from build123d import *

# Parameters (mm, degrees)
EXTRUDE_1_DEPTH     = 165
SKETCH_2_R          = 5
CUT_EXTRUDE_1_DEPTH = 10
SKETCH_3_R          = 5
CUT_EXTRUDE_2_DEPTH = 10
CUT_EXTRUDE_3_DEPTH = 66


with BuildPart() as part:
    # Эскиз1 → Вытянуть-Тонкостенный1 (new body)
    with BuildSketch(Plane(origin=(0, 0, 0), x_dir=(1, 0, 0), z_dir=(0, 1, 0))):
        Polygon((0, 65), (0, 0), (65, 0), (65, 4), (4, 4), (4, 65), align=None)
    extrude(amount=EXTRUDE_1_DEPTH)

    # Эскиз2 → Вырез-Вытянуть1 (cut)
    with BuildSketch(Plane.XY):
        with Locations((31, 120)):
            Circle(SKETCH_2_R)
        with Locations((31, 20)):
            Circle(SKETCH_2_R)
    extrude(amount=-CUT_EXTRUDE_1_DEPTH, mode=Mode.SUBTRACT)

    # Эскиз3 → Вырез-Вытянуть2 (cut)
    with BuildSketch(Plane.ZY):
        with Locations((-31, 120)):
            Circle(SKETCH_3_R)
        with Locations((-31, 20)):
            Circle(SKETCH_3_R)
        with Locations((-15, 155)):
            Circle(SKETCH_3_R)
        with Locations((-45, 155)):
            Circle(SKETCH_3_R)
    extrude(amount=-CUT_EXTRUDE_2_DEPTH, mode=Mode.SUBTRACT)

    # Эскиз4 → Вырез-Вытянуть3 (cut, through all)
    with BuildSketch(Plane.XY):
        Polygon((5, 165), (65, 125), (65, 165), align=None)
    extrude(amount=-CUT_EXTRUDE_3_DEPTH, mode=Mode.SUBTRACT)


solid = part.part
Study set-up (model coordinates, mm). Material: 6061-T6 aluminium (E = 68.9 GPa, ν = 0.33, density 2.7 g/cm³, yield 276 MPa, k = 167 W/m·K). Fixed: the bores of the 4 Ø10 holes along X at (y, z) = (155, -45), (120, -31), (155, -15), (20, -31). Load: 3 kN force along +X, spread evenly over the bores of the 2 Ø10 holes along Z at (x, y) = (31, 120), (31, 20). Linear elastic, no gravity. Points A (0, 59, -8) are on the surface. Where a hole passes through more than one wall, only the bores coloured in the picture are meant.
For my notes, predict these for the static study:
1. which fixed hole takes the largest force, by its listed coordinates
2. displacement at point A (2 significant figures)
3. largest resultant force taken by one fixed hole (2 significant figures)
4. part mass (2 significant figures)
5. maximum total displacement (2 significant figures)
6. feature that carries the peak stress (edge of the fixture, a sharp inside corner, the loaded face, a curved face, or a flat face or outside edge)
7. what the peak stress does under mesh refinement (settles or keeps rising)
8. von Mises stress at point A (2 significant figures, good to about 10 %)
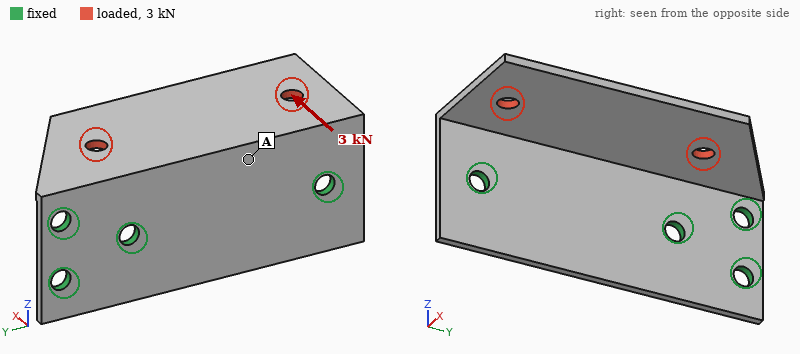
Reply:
(20, -31)
0.30 mm
1.7 kN
210 g
1.6 mm
edge of the fixture
keeps rising
44 MPa
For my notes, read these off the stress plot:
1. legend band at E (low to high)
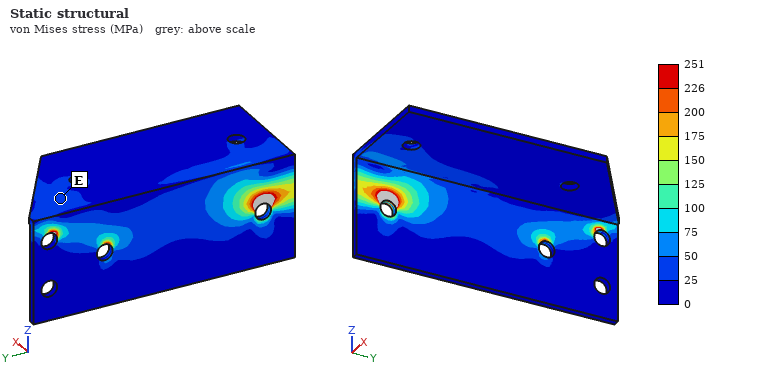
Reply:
25 to 50 MPa
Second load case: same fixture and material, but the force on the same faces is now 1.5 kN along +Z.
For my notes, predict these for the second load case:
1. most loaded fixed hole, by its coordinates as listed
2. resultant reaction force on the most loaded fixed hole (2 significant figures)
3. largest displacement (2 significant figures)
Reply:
(120, -31)
930 N
2.0 mm
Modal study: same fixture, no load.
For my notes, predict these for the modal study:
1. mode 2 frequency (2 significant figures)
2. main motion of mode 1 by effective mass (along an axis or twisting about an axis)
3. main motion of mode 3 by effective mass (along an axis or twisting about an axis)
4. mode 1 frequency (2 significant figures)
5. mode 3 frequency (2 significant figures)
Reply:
1100 Hz
along Z
along X
540 Hz
1600 Hz
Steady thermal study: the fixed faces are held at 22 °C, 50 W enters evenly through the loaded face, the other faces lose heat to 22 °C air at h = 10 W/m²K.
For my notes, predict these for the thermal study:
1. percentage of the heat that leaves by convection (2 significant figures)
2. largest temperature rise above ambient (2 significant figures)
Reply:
11 %
39 K
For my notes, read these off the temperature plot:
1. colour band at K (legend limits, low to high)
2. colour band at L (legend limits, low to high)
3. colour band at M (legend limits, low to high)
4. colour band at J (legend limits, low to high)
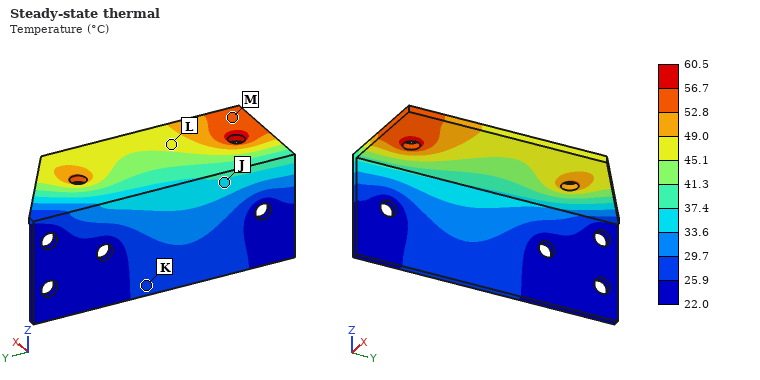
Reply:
25.9 to 29.7 °C
45.1 to 49.0 °C
52.8 to 56.7 °C
33.6 to 37.4 °C
